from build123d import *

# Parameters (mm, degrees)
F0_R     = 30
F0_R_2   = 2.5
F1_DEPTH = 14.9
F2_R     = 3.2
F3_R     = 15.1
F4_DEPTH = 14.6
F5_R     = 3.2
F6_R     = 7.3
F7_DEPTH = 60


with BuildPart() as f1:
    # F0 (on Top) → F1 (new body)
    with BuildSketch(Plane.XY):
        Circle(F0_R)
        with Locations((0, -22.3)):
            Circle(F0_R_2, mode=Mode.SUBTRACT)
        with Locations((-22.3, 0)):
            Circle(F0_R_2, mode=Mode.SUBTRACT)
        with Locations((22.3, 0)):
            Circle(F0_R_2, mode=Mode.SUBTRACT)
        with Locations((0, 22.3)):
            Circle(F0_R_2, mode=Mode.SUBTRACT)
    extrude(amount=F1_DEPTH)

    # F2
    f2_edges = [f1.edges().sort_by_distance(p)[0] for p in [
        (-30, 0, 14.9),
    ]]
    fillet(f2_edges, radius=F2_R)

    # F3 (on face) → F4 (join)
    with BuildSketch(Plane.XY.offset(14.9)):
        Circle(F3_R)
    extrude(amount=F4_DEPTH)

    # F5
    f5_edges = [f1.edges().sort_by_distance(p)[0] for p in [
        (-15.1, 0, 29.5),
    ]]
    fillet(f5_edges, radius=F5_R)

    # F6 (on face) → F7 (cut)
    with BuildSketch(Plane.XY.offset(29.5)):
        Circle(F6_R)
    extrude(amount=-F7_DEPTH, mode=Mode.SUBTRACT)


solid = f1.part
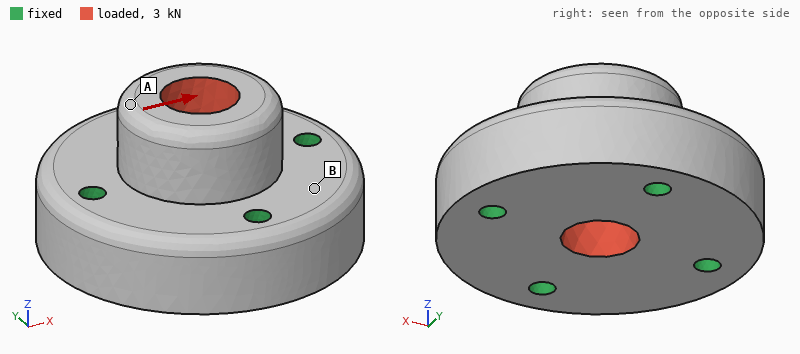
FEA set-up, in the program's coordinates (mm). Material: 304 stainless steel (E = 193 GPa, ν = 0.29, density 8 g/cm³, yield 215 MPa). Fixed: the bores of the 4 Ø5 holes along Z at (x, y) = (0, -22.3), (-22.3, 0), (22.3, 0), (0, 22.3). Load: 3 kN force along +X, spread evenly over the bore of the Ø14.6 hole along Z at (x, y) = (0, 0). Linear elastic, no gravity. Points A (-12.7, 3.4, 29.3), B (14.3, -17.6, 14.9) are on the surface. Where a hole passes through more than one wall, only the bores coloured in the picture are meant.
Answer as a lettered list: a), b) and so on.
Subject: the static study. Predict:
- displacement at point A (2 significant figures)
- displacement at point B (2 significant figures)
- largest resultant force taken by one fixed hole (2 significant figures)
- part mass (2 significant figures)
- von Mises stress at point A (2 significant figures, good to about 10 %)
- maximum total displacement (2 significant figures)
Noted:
a) 1.2 µm
b) 0.22 µm
c) 1.0 kN
d) 370 g
e) 3.4 MPa
f) 1.3 µm
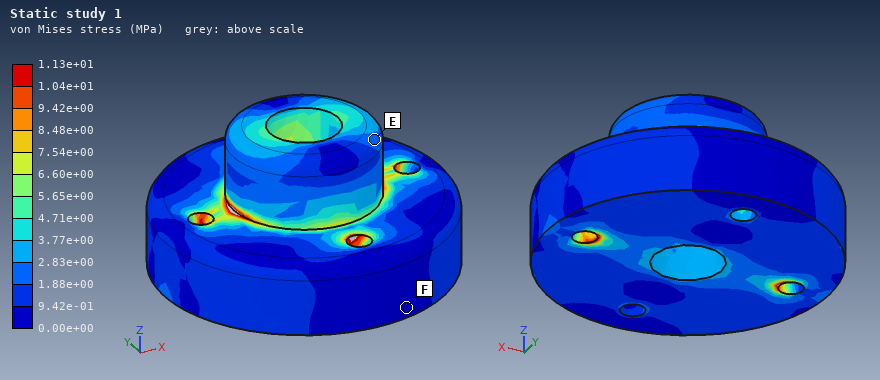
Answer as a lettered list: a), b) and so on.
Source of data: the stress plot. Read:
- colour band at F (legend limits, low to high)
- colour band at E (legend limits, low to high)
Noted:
a) 0.00e+00 to 9.42e-01 MPa
b) 1.88e+00 to 2.83e+00 MPa
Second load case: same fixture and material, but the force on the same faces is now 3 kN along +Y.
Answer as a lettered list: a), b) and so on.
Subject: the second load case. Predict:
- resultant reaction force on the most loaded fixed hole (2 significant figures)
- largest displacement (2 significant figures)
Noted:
a) 1.0 kN
b) 1.3 µm
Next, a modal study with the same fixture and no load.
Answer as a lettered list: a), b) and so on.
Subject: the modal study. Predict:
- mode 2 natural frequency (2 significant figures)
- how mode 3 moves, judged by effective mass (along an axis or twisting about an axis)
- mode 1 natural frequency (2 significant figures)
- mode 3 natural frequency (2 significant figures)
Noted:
a) 25 kHz
b) along Z
c) 25 kHz
d) 28 kHz
